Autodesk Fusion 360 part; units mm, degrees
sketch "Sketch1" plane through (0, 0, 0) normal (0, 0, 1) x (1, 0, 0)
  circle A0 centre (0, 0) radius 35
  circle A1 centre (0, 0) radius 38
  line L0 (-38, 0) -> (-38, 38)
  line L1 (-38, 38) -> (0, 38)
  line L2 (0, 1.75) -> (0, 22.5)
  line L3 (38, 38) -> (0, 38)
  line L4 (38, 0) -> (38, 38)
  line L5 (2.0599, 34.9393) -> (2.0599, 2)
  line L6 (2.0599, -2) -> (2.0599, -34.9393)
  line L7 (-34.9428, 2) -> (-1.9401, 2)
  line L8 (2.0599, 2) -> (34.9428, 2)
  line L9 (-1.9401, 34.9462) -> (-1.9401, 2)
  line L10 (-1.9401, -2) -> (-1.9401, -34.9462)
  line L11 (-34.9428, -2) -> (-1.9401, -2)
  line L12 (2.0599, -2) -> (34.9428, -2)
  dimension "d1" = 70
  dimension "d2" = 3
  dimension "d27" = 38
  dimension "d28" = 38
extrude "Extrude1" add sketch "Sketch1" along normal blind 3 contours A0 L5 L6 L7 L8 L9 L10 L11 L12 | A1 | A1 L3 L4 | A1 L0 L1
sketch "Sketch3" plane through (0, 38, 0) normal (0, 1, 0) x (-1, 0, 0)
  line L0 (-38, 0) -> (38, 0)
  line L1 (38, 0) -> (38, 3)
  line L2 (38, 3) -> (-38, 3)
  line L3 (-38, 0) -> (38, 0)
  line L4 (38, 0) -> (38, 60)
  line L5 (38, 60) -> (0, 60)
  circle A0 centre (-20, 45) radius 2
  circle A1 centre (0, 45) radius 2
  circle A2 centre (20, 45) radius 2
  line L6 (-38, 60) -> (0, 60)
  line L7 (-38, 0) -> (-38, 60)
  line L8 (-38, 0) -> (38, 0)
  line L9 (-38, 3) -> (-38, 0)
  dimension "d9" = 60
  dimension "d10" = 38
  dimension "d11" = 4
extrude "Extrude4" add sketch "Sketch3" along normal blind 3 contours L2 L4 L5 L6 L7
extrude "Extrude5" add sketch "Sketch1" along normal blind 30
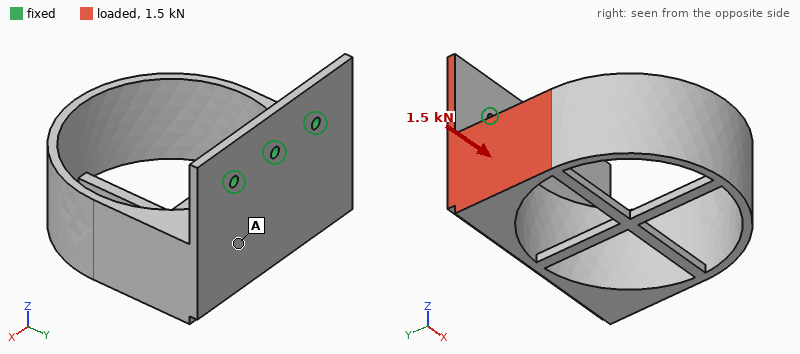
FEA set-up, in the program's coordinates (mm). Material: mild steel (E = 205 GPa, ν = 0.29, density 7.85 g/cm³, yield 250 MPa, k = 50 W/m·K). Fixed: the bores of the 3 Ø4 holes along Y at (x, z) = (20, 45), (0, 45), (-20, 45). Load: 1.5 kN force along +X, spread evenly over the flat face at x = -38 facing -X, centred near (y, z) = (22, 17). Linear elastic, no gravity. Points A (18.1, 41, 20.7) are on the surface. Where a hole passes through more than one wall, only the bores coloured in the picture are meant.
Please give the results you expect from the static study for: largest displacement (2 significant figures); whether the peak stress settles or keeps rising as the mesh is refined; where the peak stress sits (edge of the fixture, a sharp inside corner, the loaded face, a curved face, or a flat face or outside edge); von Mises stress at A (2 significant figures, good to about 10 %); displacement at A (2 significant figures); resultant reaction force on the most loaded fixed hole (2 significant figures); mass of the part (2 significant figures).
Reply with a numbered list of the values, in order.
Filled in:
1. 0.14 mm
2. keeps rising
3. edge of the fixture
4. 14 MPa
5. 0.021 mm
6. 1.3 kN
7. 420 g
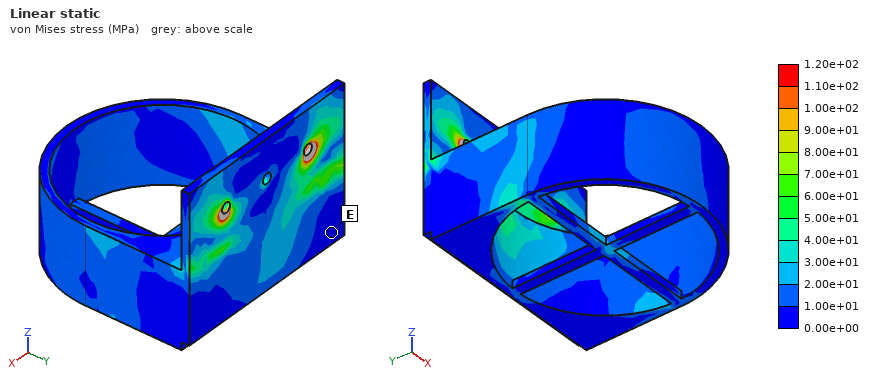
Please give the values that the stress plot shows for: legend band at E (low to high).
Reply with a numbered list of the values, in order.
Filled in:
1. 0.00e+00 to 1.00e+01 MPa
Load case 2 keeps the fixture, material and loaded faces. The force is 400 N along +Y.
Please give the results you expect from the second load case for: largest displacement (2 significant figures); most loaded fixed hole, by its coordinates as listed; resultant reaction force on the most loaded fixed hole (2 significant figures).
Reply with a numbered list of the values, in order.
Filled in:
1. 0.33 mm
2. (-20, 45)
3. 460 N
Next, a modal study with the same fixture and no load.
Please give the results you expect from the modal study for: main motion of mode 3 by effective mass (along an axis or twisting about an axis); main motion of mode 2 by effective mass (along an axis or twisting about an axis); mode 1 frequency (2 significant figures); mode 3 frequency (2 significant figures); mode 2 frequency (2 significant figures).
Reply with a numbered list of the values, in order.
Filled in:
1. along Y
2. along X
3. 290 Hz
4. 2000 Hz
5. 770 Hz
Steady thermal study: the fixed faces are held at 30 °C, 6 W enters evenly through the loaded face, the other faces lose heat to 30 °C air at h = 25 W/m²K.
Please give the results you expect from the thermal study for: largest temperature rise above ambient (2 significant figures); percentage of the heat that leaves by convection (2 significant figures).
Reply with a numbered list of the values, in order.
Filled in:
1. 13 K
2. 47 %
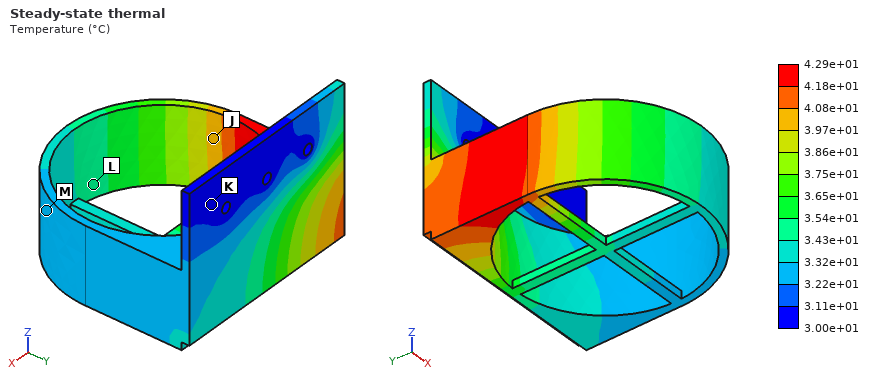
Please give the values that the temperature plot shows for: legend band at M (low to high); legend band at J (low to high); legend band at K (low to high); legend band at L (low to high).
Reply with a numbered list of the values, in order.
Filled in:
1. 3.22e+01 to 3.32e+01 °C
2. 3.97e+01 to 4.08e+01 °C
3. 3.00e+01 to 3.11e+01 °C
4. 3.43e+01 to 3.54e+01 °C
